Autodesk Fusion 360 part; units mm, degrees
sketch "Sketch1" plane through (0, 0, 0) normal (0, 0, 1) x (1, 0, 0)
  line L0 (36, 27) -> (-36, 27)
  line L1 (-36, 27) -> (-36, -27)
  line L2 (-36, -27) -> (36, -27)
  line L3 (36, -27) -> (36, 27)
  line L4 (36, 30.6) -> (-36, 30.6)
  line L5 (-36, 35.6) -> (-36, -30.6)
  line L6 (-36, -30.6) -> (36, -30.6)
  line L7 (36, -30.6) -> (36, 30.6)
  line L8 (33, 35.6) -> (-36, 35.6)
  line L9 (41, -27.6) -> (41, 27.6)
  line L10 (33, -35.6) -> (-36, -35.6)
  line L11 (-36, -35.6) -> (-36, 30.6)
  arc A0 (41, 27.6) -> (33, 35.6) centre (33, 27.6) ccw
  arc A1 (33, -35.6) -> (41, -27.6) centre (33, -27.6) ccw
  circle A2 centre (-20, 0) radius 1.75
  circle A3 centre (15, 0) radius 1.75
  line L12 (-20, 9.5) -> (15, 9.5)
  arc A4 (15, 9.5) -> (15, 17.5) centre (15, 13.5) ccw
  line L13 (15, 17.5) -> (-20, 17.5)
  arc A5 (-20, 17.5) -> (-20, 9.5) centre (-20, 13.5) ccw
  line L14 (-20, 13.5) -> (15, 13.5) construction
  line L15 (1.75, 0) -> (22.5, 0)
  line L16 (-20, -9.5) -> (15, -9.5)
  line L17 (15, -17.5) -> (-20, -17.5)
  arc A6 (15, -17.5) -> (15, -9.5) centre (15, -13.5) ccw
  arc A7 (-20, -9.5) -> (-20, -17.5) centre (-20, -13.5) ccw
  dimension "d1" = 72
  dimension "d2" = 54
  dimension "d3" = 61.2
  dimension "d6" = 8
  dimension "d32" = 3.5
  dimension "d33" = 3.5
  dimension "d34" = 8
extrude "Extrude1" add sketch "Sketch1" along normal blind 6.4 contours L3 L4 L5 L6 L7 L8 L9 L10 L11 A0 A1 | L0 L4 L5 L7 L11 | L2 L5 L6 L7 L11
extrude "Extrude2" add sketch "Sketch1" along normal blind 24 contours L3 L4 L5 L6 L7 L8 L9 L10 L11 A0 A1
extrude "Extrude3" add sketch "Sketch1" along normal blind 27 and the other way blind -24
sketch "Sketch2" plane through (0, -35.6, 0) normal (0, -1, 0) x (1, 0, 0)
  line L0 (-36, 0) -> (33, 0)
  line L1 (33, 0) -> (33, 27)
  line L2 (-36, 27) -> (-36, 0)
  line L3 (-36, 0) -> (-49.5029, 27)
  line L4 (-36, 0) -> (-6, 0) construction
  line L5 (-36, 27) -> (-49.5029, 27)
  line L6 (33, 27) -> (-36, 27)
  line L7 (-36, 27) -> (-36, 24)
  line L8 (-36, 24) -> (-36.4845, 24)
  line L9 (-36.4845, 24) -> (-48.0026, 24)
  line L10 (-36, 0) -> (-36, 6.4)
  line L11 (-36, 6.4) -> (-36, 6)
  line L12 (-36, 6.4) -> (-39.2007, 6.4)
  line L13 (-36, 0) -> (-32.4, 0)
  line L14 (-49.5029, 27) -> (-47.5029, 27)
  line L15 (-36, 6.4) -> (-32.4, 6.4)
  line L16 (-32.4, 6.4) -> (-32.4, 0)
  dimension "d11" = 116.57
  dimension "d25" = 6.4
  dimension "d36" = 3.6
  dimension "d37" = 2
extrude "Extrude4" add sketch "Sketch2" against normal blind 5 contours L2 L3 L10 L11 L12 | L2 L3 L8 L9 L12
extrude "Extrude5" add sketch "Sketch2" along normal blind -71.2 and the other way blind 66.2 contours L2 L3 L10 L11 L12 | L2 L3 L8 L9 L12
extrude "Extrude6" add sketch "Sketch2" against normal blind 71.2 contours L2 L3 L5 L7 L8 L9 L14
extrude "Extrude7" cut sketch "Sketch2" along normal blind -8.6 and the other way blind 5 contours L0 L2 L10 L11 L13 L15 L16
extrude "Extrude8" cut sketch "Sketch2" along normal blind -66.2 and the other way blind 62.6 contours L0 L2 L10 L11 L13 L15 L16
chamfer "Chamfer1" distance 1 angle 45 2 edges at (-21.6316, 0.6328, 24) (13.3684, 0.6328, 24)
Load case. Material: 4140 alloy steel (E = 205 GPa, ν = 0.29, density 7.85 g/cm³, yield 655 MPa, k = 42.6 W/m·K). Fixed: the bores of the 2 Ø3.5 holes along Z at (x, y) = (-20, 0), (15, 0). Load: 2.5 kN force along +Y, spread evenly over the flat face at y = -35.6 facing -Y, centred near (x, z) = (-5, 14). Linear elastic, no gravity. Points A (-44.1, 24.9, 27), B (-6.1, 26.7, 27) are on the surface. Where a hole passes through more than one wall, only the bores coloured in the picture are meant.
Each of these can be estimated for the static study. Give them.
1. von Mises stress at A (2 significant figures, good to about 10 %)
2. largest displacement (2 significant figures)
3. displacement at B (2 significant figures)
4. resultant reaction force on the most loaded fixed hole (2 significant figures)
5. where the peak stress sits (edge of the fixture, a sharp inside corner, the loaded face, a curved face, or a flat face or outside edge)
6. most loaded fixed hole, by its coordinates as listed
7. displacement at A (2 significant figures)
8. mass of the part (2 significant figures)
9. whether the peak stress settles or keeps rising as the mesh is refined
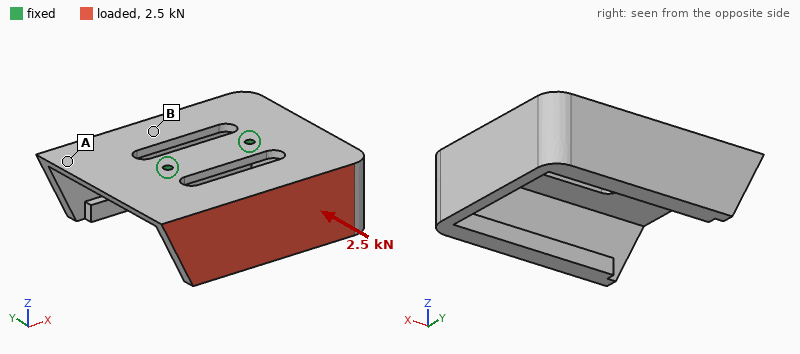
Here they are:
99 MPa
0.80 mm
0.33 mm
1.5 kN
edge of the fixture
(-20, 0)
0.23 mm
370 g
keeps rising
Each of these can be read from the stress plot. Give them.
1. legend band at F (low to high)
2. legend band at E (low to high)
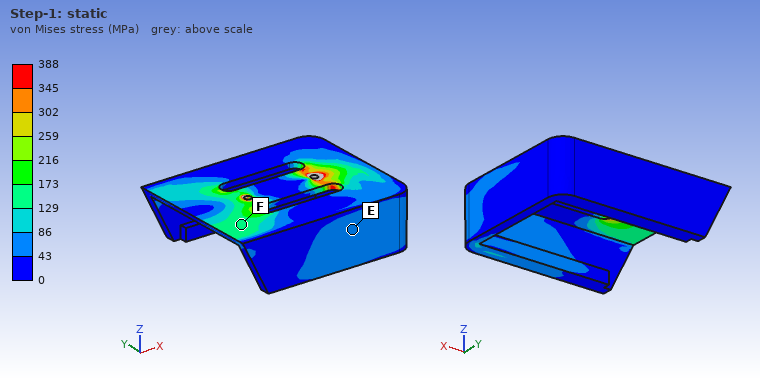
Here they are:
129 to 173 MPa
43 to 86 MPa
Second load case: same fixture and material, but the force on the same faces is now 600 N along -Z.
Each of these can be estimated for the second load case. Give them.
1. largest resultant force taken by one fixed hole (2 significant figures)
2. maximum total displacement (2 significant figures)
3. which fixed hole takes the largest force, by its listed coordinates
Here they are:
370 N
0.50 mm
(-20, 0)
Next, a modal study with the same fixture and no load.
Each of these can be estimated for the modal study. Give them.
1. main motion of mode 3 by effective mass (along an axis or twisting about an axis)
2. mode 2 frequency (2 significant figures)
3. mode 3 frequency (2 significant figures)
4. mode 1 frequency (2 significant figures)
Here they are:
along Z
950 Hz
1200 Hz
410 Hz
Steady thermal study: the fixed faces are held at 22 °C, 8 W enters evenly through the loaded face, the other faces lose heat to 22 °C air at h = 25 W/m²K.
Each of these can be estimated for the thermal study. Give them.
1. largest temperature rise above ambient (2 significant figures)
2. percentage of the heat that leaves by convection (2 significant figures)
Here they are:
26 K
66 %
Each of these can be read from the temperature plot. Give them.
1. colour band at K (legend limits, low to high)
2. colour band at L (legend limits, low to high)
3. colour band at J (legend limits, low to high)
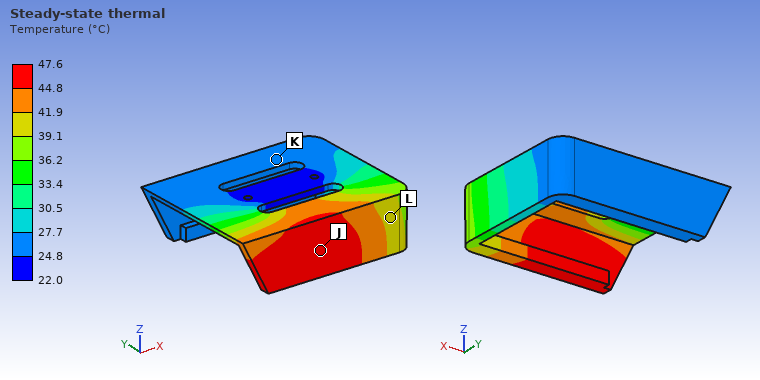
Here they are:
24.8 to 27.7 °C
39.1 to 41.9 °C
44.8 to 47.6 °C
